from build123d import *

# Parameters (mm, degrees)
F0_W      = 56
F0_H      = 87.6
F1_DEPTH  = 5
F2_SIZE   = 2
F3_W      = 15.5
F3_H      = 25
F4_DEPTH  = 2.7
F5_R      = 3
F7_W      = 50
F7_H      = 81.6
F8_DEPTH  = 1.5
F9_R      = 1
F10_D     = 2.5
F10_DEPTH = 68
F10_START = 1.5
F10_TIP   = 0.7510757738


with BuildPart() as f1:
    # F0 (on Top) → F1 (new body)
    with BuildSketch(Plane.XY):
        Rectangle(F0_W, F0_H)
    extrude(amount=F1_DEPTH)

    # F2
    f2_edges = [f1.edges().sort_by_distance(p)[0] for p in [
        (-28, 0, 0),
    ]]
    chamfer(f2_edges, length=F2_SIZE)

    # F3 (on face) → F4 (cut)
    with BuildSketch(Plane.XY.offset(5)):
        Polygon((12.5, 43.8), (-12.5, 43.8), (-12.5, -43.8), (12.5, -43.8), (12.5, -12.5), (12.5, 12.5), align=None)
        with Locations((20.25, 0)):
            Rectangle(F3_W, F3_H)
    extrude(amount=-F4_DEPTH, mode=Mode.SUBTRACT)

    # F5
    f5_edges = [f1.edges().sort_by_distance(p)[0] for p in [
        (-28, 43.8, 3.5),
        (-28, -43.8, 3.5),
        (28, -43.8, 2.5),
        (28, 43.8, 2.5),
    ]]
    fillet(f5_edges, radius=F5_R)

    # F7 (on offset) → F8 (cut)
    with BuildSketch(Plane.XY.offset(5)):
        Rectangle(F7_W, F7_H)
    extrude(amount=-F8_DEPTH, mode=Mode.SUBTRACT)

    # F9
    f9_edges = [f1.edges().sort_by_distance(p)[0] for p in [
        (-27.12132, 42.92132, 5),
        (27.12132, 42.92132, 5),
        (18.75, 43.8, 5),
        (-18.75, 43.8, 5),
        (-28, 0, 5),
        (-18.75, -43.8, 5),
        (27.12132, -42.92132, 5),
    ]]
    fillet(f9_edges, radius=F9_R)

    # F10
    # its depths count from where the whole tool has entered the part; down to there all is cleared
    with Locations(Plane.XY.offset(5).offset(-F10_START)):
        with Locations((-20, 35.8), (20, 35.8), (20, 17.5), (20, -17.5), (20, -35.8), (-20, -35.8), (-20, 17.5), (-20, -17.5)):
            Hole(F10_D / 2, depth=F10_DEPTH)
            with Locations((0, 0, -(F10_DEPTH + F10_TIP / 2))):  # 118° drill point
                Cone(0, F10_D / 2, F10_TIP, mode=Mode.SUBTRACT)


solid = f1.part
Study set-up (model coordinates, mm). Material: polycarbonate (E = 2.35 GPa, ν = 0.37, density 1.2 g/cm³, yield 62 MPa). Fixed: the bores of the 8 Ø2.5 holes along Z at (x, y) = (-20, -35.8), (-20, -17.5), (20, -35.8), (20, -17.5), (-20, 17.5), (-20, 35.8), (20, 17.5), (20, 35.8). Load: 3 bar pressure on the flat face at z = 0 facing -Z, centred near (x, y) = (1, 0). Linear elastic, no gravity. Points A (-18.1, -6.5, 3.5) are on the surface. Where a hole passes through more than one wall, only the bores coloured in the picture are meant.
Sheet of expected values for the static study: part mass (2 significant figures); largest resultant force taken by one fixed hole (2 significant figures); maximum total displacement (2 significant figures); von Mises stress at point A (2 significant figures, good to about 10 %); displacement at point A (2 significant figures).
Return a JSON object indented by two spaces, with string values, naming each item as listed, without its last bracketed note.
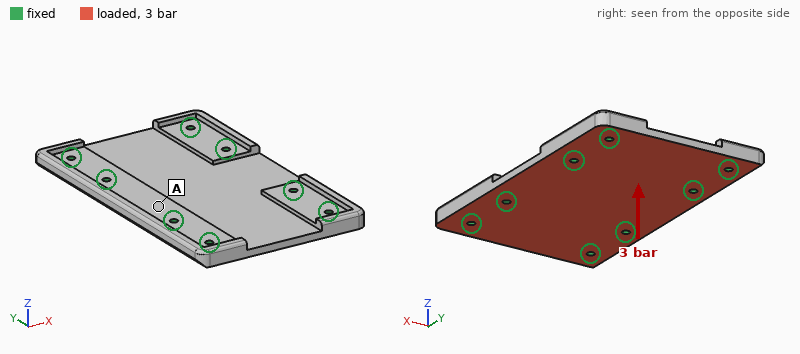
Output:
{
  "part mass": "18 g",
  "largest resultant force taken by one fixed hole": "260 N",
  "maximum total displacement": "0.83 mm",
  "von Mises stress at point A": "9.5 MPa",
  "displacement at point A": "0.23 mm"
}
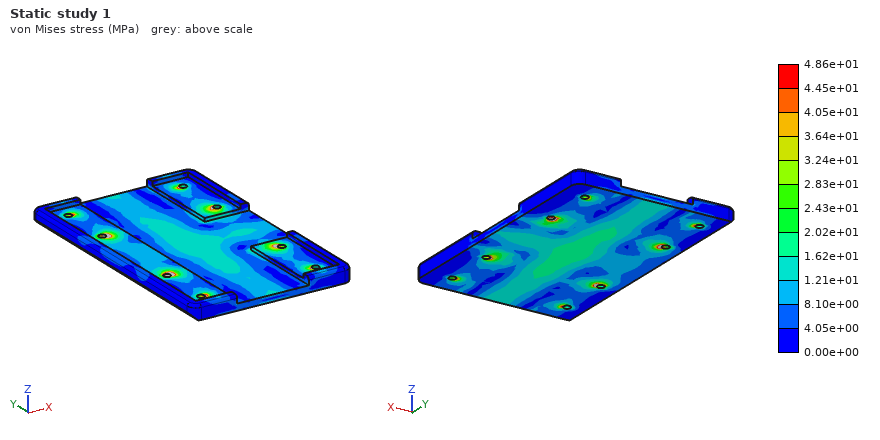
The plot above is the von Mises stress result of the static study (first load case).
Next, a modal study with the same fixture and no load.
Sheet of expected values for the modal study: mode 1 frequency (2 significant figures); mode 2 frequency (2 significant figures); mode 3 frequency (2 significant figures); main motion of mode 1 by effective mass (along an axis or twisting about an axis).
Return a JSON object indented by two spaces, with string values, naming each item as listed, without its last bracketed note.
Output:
{
  "mode 1 frequency": "2200 Hz",
  "mode 2 frequency": "2900 Hz",
  "mode 3 frequency": "3000 Hz",
  "main motion of mode 1 by effective mass": "along Z"
}
